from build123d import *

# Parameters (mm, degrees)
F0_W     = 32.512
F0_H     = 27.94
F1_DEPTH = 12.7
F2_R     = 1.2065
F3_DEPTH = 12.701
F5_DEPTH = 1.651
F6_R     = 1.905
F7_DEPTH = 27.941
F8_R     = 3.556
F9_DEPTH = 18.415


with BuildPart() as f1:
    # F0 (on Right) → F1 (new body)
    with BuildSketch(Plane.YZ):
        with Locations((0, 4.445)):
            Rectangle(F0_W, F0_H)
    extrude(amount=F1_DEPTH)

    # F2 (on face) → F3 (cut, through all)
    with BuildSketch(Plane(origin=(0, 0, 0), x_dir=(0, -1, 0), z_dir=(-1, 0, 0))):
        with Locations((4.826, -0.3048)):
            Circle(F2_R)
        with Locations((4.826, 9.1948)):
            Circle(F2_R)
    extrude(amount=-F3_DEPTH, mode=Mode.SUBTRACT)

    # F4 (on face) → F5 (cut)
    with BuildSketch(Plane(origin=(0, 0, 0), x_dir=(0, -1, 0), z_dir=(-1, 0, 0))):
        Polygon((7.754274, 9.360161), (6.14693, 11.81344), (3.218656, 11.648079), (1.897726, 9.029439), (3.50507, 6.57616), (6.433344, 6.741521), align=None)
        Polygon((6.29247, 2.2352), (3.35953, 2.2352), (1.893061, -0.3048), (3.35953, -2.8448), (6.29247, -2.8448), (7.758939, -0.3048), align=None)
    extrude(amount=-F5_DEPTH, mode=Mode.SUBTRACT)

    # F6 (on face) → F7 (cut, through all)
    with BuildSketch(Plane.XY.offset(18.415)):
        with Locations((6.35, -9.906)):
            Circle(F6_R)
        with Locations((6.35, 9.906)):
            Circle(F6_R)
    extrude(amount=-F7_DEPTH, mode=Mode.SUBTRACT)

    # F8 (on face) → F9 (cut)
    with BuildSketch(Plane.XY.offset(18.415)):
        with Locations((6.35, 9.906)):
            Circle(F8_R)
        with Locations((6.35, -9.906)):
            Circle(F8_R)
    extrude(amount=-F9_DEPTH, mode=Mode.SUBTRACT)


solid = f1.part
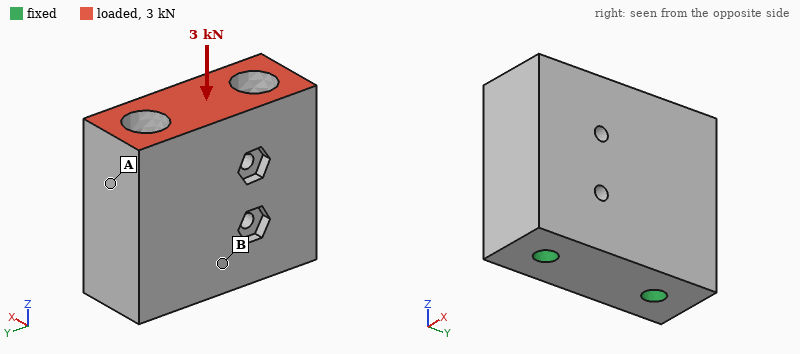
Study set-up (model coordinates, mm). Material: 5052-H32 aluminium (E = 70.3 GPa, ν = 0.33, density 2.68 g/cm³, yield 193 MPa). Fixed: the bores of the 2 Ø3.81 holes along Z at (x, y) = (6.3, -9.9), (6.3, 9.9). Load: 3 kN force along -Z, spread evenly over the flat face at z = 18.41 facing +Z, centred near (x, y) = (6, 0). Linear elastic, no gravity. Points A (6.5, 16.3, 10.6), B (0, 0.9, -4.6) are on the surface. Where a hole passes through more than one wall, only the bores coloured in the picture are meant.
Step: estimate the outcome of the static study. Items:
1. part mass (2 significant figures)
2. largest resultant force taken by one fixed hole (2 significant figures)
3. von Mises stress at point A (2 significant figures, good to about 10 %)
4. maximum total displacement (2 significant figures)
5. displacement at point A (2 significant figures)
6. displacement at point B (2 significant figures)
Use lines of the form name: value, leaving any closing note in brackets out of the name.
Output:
part mass: 26 g
largest resultant force taken by one fixed hole: 1.5 kN
von Mises stress at point A: 9.1 MPa
maximum total displacement: 4.5 µm
displacement at point A: 2.8 µm
displacement at point B: 1.8 µm
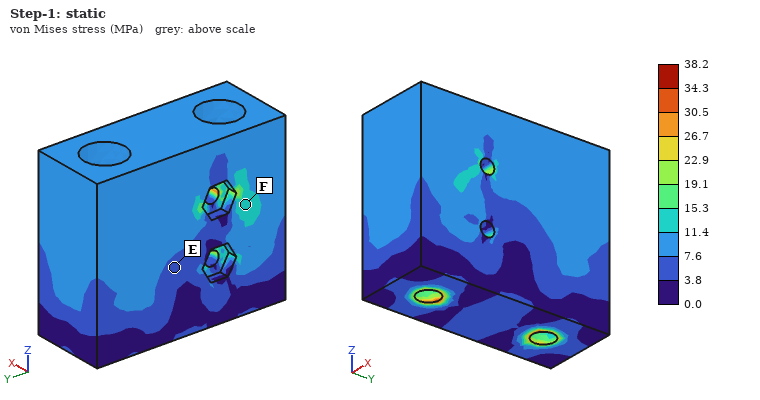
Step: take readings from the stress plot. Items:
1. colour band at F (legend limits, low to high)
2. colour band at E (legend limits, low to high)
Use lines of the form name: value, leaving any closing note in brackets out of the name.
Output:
colour band at F: 11.4 to 15.3 MPa
colour band at E: 3.8 to 7.6 MPa
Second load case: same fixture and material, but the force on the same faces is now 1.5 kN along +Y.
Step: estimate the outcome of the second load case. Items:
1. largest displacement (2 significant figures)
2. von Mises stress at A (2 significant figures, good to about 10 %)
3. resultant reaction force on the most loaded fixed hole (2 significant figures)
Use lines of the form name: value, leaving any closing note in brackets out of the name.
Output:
largest displacement: 13 µm
von Mises stress at A: 8.5 MPa
resultant reaction force on the most loaded fixed hole: 1.6 kN
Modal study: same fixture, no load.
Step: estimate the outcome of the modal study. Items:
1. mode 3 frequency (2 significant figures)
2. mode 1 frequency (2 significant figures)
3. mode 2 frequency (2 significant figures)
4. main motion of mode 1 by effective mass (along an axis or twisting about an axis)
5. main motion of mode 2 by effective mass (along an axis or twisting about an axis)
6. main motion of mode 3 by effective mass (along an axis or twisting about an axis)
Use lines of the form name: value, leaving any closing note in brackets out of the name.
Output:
mode 3 frequency: 24 kHz
mode 1 frequency: 12 kHz
mode 2 frequency: 23 kHz
main motion of mode 1 by effective mass: along X
main motion of mode 2 by effective mass: along Y
main motion of mode 3 by effective mass: twisting about Z
